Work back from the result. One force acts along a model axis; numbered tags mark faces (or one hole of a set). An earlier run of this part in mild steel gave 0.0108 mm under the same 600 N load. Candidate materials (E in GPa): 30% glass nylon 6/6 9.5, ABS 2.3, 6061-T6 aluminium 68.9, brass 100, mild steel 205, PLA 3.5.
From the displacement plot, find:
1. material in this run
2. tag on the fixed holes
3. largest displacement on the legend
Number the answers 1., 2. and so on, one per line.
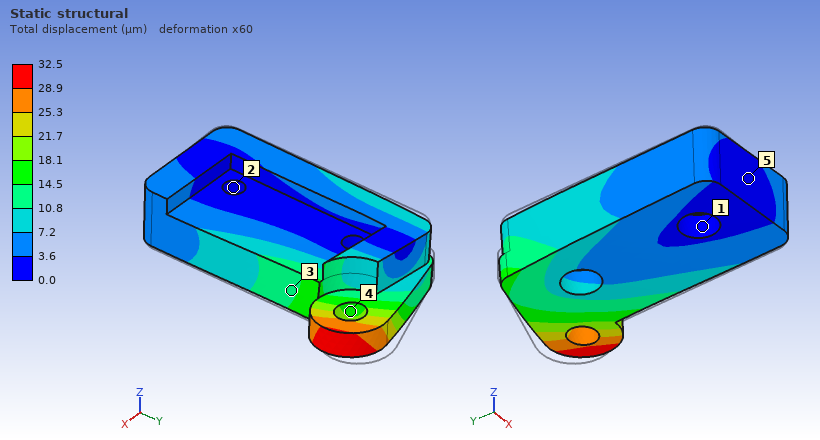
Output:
1. 6061-T6 aluminium
2. 2
3. 32.5 µm
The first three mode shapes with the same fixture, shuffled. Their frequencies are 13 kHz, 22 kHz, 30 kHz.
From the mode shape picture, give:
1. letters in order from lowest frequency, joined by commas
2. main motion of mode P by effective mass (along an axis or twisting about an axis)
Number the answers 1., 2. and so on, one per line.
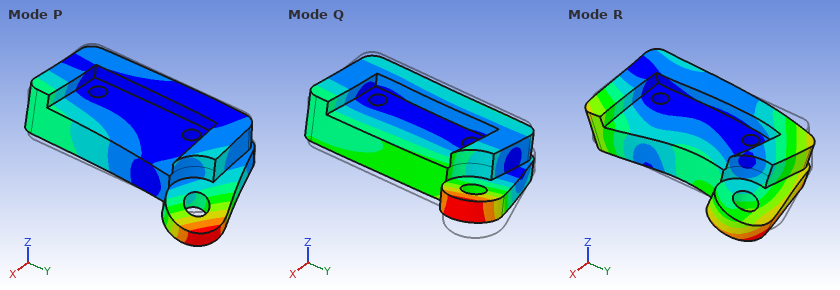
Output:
1. Q, P, R
2. twisting about X
